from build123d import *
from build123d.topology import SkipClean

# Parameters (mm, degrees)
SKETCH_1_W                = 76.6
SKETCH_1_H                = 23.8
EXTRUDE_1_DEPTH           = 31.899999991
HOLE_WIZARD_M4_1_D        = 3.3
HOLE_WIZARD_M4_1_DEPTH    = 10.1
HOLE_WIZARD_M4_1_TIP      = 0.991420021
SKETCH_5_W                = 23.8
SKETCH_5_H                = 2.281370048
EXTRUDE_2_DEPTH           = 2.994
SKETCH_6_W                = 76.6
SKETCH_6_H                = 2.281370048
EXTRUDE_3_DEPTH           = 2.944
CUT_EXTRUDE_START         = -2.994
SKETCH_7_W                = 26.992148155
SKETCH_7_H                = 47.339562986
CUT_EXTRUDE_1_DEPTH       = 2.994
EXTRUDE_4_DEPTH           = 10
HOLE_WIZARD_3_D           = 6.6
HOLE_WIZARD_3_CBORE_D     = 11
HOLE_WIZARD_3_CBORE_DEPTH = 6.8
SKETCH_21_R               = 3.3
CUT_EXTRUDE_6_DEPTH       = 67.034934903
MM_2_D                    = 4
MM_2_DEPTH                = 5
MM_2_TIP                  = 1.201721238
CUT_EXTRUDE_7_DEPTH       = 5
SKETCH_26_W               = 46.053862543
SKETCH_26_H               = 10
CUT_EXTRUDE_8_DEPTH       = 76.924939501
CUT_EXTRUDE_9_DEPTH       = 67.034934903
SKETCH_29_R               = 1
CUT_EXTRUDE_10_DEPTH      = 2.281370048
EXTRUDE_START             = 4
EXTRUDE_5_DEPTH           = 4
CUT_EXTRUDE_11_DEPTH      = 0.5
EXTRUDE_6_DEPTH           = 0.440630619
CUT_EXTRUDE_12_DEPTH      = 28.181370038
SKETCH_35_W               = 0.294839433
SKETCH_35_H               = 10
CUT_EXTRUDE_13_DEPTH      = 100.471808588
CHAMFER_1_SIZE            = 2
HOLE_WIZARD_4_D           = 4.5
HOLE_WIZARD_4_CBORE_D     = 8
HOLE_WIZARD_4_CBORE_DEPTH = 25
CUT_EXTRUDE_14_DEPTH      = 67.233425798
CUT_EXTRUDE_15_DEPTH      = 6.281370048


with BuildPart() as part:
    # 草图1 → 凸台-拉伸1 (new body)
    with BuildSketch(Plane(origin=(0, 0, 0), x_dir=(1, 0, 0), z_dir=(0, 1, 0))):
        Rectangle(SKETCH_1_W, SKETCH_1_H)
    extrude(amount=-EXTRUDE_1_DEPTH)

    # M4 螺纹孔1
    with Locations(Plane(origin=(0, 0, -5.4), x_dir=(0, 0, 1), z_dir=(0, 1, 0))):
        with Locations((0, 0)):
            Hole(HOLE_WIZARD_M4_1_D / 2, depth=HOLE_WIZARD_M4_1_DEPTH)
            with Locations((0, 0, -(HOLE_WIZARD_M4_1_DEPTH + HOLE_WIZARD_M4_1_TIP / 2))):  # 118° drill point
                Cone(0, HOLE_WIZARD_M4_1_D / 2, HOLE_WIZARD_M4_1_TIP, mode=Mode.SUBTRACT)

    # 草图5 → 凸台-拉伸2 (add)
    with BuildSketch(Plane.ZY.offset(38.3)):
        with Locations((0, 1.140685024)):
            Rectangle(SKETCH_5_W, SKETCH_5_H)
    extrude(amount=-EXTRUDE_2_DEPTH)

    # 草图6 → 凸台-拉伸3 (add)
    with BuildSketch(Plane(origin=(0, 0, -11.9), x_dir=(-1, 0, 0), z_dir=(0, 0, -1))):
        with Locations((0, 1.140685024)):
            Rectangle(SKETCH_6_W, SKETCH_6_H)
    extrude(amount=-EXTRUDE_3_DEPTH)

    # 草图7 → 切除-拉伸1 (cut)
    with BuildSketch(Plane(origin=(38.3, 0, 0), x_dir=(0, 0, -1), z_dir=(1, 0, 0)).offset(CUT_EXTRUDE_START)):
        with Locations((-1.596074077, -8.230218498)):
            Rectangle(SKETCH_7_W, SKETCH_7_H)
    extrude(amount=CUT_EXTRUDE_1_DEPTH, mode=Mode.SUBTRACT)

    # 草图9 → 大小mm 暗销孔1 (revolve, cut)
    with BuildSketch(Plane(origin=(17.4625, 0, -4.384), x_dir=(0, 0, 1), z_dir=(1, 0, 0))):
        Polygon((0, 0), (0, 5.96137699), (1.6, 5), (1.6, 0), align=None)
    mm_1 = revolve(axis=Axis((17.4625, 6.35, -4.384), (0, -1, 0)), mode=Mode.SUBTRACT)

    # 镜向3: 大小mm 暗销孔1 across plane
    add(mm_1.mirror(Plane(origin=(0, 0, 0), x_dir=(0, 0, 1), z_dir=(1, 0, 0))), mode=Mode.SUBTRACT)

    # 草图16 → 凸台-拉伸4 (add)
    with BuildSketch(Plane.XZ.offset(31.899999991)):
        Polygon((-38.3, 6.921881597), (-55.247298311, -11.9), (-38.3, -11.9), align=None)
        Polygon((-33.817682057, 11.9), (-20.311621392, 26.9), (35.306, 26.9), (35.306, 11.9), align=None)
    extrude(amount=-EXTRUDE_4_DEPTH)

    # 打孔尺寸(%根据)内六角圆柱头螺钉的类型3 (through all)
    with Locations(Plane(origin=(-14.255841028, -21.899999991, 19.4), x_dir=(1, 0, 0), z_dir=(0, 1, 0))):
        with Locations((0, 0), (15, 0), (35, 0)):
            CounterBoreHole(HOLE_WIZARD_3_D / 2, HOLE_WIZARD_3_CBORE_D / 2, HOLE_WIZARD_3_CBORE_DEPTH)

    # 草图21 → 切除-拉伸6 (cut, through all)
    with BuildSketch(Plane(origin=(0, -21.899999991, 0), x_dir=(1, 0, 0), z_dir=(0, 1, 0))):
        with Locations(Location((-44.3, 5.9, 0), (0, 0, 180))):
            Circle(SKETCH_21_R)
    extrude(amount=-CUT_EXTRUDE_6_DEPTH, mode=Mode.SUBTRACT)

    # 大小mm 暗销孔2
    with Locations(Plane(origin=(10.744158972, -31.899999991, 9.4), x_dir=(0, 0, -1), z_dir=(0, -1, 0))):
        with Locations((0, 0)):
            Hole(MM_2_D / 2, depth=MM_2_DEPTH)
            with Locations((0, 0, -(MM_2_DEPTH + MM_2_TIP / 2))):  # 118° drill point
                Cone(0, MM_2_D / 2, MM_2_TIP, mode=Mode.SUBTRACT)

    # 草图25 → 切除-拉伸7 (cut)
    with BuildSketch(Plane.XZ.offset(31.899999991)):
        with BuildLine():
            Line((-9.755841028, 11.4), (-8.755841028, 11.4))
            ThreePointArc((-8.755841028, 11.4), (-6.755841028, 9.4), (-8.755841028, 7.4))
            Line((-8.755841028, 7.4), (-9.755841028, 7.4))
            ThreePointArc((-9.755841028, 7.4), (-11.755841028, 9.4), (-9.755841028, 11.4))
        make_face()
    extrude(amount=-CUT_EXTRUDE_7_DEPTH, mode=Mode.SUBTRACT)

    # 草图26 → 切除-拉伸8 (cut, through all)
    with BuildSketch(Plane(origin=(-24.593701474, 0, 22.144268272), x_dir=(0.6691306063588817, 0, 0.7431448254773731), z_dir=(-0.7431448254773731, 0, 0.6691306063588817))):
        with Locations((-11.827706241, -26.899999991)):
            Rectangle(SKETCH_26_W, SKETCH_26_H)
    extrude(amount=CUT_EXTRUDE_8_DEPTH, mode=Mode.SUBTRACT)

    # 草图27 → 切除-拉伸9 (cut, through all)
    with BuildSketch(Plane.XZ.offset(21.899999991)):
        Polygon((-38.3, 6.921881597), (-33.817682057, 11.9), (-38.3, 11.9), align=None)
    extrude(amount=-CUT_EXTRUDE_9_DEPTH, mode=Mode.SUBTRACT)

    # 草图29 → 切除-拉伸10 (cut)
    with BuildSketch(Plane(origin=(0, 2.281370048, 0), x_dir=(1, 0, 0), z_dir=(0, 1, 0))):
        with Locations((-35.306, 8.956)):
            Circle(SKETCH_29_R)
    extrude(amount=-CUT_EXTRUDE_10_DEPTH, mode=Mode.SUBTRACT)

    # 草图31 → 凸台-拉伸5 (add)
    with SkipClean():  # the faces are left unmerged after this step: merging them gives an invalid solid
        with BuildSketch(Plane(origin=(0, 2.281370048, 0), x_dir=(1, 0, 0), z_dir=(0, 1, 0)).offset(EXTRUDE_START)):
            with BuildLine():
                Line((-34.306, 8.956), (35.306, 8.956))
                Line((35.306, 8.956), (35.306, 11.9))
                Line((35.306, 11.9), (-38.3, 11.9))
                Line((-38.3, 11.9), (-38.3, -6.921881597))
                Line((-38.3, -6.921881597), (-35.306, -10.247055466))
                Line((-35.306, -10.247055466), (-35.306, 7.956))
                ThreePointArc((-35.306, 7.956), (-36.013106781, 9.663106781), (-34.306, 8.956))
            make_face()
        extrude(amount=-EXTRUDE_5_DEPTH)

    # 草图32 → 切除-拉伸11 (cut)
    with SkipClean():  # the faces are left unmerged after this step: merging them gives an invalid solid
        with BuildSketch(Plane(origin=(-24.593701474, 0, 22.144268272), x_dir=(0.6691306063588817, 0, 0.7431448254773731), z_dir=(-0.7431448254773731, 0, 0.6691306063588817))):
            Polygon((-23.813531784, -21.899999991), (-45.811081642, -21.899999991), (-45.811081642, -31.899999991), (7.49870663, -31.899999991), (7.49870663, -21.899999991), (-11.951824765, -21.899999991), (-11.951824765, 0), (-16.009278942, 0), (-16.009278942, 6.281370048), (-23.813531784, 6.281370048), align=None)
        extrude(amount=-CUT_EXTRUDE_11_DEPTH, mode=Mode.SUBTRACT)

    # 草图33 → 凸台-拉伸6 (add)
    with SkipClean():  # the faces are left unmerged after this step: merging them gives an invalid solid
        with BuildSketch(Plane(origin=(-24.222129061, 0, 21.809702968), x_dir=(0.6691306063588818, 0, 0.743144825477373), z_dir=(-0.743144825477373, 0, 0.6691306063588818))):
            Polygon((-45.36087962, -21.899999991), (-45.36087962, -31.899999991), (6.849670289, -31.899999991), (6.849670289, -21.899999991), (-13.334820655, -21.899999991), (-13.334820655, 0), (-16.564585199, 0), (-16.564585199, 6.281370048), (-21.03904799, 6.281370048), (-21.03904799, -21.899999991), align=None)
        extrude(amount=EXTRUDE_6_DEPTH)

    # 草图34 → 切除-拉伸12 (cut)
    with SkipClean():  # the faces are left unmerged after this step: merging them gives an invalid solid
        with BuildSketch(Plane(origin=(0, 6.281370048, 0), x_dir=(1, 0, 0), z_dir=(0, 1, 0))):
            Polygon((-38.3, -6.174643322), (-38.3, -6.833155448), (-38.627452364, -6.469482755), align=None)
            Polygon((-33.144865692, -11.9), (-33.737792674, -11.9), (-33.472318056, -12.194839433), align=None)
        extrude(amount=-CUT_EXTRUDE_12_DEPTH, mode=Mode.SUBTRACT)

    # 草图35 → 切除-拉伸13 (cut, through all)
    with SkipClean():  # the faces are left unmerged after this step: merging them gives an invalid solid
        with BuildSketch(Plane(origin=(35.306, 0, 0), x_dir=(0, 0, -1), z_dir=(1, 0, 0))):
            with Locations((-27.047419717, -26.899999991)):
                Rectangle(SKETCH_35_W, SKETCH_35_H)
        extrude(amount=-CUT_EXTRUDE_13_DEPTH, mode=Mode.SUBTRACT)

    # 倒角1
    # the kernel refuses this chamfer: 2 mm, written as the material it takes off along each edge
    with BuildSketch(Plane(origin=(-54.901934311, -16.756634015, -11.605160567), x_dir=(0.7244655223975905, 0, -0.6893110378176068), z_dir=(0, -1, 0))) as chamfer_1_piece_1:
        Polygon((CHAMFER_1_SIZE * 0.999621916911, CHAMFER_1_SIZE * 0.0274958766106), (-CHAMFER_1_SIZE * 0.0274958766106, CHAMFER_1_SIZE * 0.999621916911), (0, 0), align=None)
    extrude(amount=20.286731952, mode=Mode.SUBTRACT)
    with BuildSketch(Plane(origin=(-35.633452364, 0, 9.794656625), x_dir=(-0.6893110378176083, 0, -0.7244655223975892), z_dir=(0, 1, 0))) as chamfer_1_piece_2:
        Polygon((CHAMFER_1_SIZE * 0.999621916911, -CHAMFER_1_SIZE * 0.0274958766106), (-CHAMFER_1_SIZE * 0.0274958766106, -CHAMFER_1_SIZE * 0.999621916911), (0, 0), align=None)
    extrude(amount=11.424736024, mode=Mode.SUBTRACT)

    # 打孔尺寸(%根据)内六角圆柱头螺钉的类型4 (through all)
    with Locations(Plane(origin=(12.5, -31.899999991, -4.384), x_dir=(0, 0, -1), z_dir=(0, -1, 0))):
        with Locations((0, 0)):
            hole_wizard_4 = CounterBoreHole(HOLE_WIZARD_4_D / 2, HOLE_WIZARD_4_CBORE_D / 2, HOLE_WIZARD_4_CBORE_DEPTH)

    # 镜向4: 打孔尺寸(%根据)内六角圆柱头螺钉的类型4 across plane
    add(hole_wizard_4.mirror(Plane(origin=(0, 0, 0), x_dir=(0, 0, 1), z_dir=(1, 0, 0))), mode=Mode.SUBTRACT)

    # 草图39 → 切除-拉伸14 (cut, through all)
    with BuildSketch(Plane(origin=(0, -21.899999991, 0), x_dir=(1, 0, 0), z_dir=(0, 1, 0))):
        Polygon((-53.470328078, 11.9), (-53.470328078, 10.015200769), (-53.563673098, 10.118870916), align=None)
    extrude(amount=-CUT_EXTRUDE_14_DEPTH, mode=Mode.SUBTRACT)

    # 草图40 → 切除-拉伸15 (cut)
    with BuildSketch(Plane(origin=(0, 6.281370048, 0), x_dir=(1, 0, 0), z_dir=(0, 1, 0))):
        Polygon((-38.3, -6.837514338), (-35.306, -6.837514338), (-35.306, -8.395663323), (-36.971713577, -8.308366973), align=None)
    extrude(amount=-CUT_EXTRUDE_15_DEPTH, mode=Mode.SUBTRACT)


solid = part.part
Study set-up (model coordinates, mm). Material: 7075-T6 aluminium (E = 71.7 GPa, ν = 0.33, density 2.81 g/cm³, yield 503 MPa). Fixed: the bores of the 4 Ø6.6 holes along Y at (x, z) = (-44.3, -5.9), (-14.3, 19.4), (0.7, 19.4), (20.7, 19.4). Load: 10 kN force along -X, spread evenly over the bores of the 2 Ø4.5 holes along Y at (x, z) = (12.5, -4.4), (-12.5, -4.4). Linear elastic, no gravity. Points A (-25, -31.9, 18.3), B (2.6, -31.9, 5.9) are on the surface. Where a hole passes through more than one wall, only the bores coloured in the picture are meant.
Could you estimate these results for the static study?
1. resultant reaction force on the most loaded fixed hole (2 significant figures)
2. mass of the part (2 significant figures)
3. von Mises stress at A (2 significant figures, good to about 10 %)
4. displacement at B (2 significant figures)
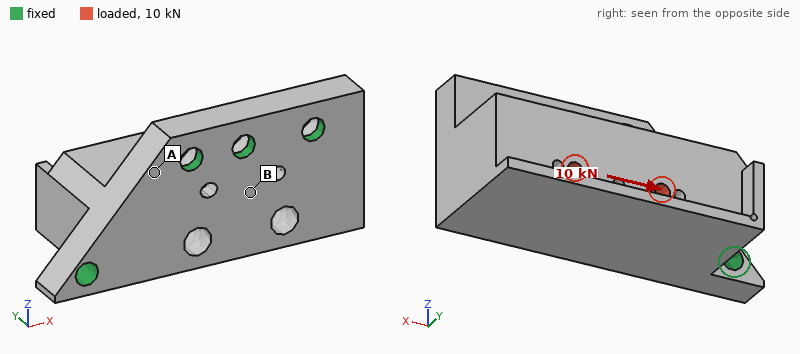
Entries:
5.8 kN
180 g
37 MPa
0.028 mm
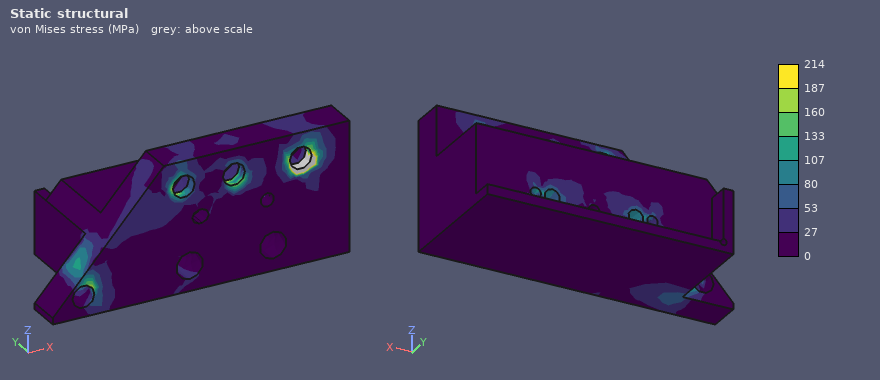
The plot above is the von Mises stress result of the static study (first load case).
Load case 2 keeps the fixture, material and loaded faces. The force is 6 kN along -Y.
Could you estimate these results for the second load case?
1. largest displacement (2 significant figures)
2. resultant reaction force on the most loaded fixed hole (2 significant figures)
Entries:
0.19 mm
4.1 kN
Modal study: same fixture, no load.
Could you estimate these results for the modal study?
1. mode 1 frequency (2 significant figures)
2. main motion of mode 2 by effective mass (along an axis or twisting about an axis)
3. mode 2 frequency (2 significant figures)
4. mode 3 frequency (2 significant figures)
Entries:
3000 Hz
along X
9900 Hz
10 kHz
